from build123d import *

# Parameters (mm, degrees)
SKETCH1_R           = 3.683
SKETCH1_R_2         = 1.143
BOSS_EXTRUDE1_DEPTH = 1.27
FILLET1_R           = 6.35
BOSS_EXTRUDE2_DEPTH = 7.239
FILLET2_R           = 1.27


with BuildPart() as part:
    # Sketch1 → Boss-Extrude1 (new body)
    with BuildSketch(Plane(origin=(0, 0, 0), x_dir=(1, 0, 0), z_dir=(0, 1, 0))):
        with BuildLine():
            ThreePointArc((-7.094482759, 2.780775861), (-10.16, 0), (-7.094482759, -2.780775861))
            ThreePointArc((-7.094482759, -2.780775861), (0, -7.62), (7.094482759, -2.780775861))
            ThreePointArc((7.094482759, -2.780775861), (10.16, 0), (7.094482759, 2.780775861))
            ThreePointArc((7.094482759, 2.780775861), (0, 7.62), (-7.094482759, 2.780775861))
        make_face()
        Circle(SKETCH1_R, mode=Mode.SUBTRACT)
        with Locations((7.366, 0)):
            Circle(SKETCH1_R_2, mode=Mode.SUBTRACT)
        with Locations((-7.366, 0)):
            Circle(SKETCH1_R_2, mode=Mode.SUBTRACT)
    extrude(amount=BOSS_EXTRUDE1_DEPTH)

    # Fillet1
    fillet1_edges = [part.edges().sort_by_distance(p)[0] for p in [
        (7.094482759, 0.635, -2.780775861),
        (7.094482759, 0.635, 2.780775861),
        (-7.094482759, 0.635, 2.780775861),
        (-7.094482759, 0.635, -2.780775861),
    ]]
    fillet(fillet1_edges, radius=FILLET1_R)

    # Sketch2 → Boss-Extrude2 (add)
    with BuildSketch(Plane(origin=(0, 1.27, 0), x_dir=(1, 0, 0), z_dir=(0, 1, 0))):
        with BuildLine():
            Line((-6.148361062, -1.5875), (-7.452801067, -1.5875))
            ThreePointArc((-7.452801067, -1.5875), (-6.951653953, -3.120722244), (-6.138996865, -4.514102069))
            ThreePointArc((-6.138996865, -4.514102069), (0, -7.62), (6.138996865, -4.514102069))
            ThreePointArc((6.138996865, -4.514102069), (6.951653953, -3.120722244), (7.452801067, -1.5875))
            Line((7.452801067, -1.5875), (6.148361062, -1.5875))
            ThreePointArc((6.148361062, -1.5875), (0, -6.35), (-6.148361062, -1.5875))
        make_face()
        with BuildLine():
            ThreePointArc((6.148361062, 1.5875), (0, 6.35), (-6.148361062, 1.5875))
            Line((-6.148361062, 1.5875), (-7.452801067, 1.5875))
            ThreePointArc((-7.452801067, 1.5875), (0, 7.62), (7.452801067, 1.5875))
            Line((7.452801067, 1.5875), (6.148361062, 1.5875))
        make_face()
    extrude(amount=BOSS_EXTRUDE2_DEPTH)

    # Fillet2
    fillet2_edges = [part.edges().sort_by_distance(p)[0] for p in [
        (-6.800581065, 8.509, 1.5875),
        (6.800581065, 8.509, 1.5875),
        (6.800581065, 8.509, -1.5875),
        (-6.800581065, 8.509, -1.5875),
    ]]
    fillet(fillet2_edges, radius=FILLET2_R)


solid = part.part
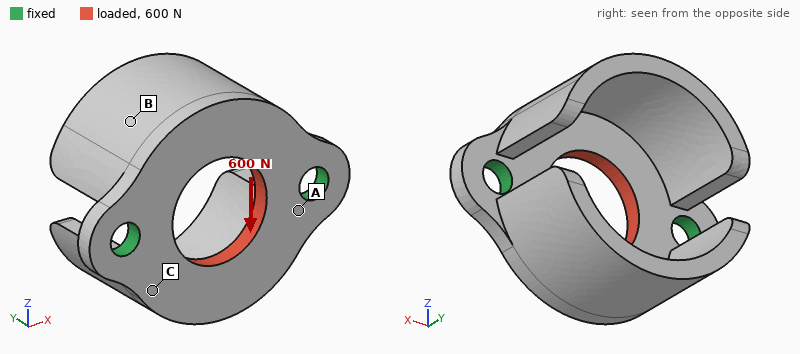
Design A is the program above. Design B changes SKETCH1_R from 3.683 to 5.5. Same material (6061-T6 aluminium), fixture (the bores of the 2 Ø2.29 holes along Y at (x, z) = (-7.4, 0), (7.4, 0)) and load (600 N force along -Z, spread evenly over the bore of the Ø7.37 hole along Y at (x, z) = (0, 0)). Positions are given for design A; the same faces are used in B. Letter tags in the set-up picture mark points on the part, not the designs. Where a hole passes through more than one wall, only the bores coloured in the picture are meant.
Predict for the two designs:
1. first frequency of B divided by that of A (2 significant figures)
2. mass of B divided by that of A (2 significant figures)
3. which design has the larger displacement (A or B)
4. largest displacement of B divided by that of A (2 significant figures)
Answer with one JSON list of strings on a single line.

["0.94", "0.88", "B", "1.4"]
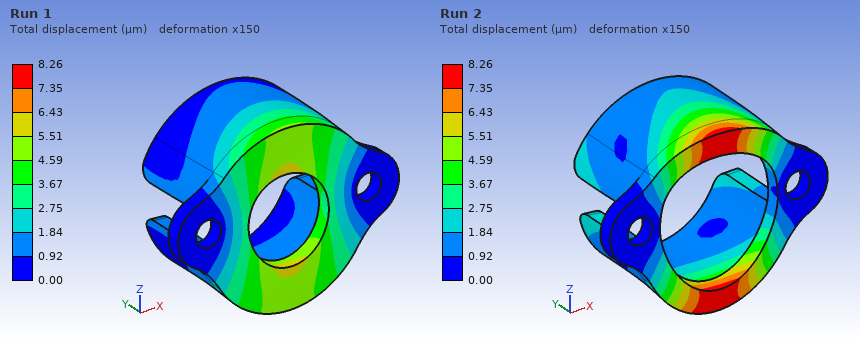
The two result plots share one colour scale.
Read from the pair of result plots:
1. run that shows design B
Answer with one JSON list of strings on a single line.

["Run 2"]
